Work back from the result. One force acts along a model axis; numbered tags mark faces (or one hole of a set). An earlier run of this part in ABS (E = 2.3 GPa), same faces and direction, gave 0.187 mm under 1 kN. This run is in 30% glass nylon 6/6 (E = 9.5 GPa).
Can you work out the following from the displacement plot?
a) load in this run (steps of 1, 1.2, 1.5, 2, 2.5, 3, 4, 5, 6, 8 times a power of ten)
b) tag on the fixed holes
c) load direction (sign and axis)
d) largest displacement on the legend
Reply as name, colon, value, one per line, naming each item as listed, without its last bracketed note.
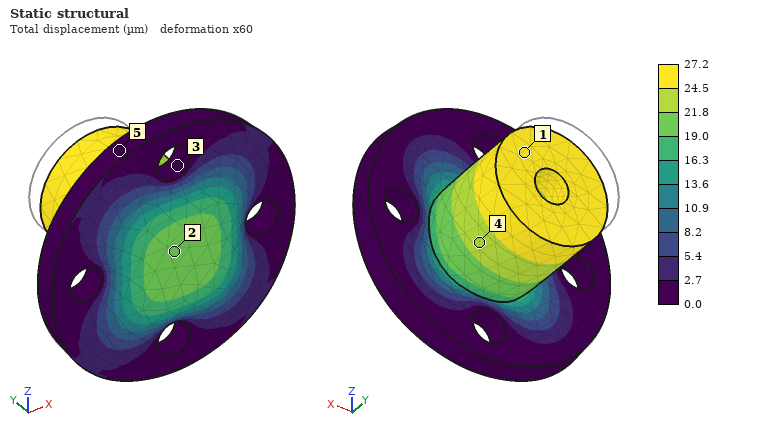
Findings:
load in this run: 600 N
tag on the fixed holes: 3
load direction: -Y
largest displacement on the legend: 27.2 µm
